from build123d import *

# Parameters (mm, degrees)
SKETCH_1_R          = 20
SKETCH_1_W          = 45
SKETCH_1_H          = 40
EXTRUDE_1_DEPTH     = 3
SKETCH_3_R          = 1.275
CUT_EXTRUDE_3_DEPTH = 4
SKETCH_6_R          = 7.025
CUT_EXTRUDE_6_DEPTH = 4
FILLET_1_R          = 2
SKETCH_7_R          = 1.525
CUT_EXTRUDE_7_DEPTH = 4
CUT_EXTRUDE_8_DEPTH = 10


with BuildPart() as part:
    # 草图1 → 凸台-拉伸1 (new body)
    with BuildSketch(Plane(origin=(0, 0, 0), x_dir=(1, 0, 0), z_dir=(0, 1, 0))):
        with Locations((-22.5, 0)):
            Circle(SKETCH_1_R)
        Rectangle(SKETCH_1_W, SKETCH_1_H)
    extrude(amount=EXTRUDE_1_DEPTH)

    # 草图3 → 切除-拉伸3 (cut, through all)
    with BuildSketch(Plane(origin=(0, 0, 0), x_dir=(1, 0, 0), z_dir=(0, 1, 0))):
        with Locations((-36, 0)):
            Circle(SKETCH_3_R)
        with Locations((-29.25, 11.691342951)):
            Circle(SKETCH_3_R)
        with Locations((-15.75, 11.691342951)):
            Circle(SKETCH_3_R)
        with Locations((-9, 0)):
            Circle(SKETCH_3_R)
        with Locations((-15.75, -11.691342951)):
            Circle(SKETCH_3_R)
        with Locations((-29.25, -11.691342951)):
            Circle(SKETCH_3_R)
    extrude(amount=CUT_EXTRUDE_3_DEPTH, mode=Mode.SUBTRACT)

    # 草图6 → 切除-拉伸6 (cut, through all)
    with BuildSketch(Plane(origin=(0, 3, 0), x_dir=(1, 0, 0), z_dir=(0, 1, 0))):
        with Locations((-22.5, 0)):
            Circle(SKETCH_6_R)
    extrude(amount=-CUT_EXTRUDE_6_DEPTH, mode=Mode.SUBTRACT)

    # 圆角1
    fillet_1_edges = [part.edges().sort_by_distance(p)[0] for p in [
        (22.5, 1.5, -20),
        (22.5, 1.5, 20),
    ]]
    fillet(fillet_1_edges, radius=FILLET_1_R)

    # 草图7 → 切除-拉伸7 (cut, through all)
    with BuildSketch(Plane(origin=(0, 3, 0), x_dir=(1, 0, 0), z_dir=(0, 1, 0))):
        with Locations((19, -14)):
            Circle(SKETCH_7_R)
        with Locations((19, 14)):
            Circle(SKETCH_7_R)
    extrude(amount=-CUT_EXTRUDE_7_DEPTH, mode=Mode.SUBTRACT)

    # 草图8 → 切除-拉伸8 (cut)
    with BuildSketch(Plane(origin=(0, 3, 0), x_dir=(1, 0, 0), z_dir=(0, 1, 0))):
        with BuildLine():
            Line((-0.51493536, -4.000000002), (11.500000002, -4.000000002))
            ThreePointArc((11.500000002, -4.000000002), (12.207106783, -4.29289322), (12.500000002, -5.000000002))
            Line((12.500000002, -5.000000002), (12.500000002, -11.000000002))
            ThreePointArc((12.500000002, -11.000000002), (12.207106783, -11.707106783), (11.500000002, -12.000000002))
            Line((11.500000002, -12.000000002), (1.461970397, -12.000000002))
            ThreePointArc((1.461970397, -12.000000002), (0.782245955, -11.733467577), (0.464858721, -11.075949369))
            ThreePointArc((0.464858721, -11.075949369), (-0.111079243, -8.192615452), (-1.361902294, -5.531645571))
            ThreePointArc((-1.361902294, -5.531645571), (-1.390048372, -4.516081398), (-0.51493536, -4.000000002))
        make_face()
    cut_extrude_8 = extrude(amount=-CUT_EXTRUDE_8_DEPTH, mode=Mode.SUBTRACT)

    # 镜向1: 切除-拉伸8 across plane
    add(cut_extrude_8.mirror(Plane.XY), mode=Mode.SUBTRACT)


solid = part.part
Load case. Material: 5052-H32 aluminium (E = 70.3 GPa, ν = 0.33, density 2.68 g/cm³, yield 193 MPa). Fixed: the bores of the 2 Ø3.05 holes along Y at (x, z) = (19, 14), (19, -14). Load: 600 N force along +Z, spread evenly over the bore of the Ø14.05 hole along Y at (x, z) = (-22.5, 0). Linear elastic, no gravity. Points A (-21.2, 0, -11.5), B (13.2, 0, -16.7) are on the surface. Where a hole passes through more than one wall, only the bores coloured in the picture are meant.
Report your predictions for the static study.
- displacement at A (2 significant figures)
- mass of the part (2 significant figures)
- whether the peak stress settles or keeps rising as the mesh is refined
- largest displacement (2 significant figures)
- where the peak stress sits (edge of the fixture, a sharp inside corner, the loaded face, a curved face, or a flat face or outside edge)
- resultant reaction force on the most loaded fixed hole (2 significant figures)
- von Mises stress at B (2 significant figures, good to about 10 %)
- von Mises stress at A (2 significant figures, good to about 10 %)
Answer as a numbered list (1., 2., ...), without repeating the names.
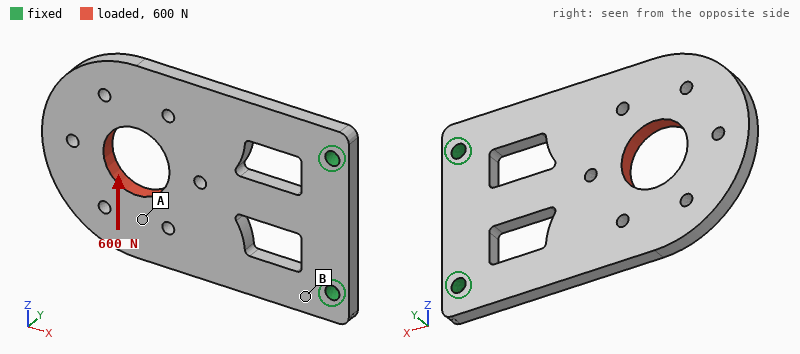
1. 46 µm
2. 16 g
3. keeps rising
4. 62 µm
5. edge of the fixture
6. 850 N
7. 35 MPa
8. 12 MPa
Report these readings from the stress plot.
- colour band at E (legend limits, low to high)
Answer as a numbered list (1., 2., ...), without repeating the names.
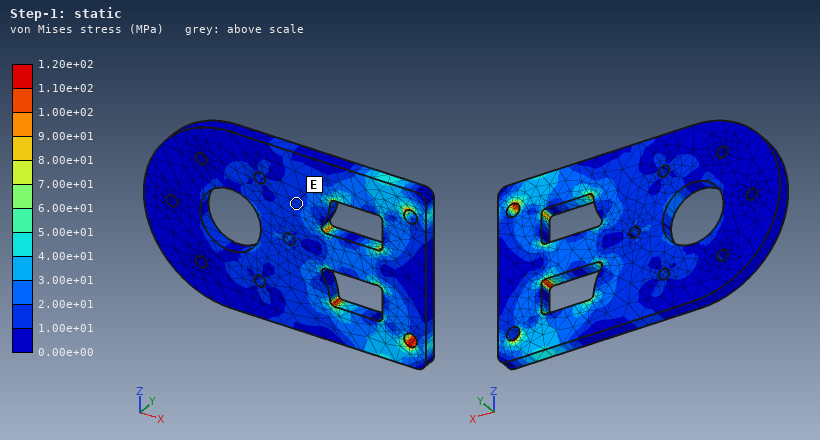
1. 1.00e+01 to 2.00e+01 MPa
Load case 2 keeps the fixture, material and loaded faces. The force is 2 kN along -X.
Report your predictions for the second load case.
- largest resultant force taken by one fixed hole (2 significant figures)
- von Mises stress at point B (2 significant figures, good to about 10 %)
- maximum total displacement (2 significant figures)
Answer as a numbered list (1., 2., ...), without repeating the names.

1. 1.0 kN
2. 34 MPa
3. 22 µm
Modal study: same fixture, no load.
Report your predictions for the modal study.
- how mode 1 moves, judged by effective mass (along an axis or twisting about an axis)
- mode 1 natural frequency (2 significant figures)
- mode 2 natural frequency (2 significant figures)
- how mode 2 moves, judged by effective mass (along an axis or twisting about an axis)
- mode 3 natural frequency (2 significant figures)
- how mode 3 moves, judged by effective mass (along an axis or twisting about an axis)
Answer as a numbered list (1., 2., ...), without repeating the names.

1. along Y
2. 650 Hz
3. 2300 Hz
4. twisting about X
5. 4000 Hz
6. along Y
